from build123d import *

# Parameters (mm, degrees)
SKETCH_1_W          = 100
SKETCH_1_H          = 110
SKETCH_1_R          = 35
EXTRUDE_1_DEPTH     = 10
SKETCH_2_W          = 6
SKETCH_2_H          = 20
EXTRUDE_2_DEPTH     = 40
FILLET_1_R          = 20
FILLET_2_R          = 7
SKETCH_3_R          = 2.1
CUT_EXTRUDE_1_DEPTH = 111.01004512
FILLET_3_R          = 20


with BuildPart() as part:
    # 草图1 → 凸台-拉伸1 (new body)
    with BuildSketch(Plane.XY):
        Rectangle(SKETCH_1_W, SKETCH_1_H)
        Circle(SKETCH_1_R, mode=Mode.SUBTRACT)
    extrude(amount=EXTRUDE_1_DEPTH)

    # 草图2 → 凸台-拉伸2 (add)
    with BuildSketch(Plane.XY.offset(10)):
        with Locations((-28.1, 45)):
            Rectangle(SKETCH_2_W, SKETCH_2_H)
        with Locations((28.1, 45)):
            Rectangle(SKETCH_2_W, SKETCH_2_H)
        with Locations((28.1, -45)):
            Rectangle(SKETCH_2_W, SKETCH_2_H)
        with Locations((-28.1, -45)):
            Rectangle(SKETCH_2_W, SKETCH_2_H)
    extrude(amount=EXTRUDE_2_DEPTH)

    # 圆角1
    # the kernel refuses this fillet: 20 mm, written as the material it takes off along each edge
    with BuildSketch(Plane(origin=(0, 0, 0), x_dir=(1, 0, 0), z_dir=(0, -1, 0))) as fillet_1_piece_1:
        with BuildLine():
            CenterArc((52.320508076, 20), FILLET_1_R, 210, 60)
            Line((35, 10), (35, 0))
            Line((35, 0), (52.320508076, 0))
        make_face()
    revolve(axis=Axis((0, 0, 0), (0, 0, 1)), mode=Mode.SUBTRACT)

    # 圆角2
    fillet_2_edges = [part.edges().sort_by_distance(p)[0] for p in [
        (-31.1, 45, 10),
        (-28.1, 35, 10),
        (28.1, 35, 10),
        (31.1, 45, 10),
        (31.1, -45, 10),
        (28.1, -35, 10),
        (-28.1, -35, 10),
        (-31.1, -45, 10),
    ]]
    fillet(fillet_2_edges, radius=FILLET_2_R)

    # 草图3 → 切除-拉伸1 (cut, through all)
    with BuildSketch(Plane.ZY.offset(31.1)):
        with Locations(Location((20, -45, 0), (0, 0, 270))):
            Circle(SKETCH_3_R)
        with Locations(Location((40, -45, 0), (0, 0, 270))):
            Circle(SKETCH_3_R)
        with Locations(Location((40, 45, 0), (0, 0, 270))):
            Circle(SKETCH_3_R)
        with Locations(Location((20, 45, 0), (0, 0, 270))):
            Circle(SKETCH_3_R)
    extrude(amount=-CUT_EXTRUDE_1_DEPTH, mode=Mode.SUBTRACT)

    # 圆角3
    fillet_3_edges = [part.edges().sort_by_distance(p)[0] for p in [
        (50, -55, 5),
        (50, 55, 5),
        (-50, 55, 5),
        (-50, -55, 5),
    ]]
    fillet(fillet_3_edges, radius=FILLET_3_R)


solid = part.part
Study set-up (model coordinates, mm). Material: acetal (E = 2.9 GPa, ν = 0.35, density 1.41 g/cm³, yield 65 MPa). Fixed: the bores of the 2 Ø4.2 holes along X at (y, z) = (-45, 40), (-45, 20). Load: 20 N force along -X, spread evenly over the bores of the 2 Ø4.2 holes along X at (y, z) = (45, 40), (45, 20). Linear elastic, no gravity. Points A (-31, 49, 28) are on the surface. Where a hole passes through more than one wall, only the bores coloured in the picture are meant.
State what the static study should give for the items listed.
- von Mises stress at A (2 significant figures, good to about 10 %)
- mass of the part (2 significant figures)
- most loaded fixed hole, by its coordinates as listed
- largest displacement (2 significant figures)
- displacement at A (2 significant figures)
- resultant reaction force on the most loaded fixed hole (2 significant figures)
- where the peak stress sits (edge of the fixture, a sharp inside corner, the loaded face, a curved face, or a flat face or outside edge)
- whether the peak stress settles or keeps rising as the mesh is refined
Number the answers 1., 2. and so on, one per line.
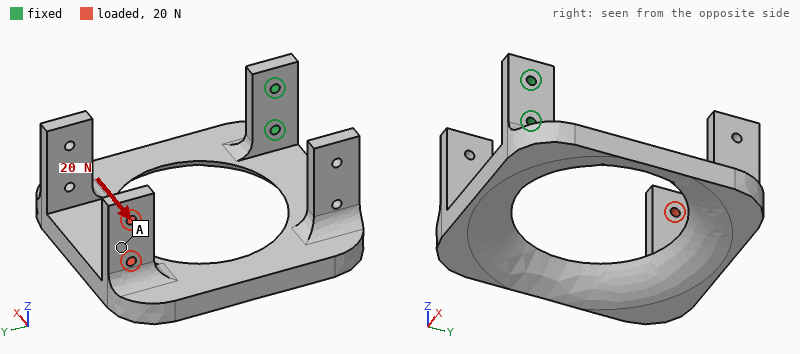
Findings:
1. 1.0 MPa
2. 110 g
3. (-45, 20)
4. 1.7 mm
5. 1.4 mm
6. 17 N
7. edge of the fixture
8. keeps rising
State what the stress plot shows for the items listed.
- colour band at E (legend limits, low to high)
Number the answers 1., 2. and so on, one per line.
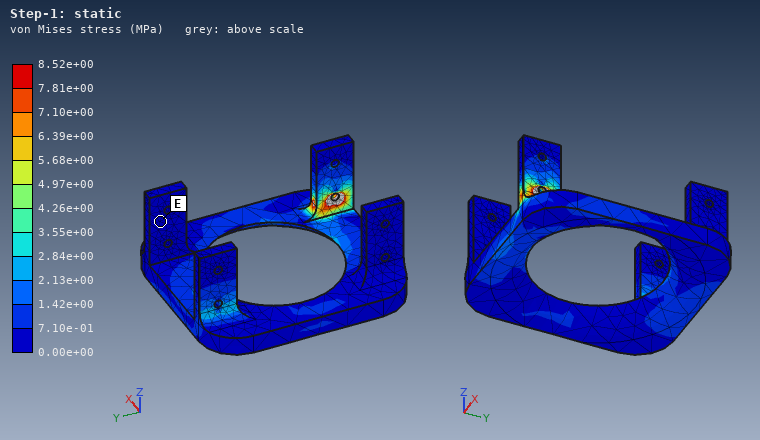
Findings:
1. 0.00e+00 to 7.10e-01 MPa
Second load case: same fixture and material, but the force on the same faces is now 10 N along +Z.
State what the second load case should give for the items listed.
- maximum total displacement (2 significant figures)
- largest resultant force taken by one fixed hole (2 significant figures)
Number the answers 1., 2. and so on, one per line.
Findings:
1. 1.6 mm
2. 33 N
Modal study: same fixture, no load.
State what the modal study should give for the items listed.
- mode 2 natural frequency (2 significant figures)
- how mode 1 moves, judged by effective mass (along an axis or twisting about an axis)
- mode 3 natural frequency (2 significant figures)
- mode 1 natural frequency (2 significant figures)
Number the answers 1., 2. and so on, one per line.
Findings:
1. 84 Hz
2. along Z
3. 130 Hz
4. 73 Hz
